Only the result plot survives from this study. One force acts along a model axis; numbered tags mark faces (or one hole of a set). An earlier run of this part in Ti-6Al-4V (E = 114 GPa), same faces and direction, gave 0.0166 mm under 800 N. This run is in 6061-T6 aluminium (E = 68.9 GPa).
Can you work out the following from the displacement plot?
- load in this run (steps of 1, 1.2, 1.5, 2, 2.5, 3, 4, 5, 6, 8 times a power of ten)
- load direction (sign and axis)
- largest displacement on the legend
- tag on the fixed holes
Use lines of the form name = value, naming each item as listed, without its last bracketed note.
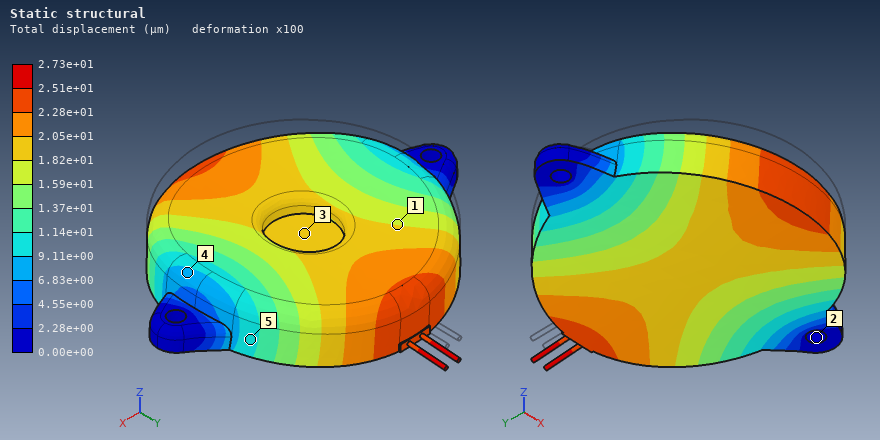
load in this run = 800 N
load direction = -Z
largest displacement on the legend = 2.73e+01 µm
tag on the fixed holes = 2
